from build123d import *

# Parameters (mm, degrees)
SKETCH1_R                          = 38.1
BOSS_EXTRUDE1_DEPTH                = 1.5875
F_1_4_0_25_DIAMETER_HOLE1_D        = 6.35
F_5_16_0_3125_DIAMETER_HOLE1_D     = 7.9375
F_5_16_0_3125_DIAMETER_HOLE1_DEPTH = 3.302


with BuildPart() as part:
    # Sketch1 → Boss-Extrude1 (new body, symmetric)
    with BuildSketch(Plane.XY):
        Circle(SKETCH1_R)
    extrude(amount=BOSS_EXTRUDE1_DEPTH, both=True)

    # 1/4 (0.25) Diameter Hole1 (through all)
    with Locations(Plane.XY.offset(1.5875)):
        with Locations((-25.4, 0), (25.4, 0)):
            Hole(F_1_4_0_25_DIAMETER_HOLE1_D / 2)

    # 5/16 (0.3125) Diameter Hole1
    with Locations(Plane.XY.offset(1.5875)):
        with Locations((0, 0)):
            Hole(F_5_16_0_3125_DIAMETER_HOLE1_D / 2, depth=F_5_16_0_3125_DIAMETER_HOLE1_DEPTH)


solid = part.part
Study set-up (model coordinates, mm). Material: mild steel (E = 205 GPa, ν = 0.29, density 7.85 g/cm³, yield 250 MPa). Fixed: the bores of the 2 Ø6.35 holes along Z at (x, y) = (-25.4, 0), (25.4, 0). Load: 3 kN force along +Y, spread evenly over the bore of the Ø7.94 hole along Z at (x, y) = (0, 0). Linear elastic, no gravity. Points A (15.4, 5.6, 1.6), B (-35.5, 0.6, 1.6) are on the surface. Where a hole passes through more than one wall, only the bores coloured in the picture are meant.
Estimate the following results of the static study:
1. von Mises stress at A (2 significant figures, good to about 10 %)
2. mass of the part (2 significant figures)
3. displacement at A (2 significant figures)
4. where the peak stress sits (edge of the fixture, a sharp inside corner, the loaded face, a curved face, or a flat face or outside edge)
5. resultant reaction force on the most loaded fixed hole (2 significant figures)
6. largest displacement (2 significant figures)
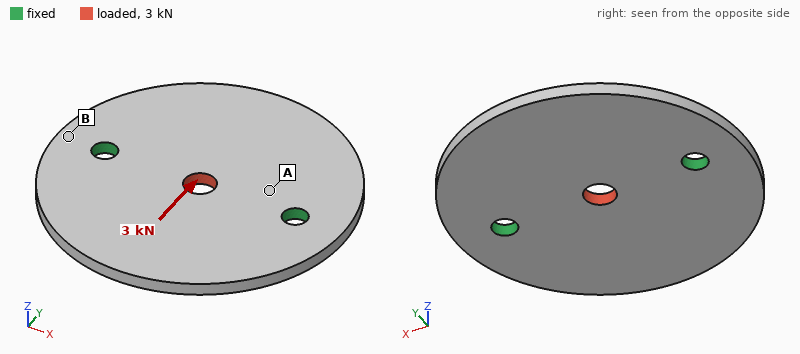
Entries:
17 MPa
110 g
1.7 µm
edge of the fixture
1.5 kN
4.2 µm
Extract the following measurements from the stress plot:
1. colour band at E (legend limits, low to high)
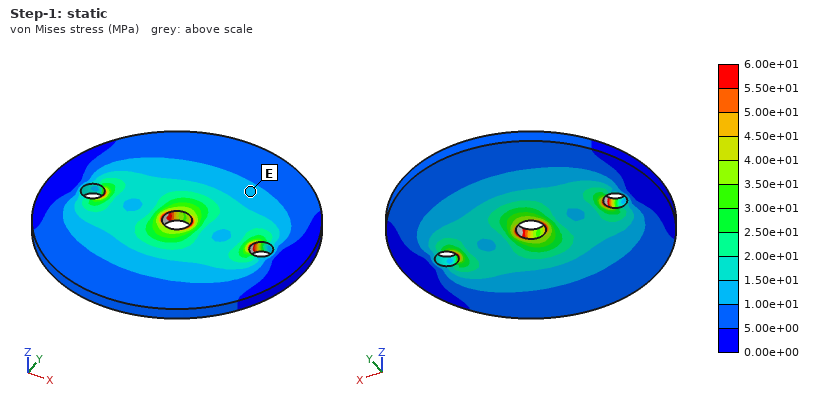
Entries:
1.00e+01 to 1.50e+01 MPa
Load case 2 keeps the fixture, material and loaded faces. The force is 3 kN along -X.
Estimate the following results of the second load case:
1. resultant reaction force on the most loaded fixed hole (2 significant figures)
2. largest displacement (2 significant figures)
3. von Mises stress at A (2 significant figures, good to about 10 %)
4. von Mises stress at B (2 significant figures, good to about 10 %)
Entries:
1.5 kN
3.1 µm
20 MPa
7.1 MPa
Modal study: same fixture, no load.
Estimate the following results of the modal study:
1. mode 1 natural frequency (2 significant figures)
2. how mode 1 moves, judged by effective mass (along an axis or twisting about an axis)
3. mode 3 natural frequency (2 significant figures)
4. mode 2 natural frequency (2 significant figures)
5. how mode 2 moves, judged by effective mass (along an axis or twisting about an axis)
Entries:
2000 Hz
twisting about X
5000 Hz
2300 Hz
along Z
